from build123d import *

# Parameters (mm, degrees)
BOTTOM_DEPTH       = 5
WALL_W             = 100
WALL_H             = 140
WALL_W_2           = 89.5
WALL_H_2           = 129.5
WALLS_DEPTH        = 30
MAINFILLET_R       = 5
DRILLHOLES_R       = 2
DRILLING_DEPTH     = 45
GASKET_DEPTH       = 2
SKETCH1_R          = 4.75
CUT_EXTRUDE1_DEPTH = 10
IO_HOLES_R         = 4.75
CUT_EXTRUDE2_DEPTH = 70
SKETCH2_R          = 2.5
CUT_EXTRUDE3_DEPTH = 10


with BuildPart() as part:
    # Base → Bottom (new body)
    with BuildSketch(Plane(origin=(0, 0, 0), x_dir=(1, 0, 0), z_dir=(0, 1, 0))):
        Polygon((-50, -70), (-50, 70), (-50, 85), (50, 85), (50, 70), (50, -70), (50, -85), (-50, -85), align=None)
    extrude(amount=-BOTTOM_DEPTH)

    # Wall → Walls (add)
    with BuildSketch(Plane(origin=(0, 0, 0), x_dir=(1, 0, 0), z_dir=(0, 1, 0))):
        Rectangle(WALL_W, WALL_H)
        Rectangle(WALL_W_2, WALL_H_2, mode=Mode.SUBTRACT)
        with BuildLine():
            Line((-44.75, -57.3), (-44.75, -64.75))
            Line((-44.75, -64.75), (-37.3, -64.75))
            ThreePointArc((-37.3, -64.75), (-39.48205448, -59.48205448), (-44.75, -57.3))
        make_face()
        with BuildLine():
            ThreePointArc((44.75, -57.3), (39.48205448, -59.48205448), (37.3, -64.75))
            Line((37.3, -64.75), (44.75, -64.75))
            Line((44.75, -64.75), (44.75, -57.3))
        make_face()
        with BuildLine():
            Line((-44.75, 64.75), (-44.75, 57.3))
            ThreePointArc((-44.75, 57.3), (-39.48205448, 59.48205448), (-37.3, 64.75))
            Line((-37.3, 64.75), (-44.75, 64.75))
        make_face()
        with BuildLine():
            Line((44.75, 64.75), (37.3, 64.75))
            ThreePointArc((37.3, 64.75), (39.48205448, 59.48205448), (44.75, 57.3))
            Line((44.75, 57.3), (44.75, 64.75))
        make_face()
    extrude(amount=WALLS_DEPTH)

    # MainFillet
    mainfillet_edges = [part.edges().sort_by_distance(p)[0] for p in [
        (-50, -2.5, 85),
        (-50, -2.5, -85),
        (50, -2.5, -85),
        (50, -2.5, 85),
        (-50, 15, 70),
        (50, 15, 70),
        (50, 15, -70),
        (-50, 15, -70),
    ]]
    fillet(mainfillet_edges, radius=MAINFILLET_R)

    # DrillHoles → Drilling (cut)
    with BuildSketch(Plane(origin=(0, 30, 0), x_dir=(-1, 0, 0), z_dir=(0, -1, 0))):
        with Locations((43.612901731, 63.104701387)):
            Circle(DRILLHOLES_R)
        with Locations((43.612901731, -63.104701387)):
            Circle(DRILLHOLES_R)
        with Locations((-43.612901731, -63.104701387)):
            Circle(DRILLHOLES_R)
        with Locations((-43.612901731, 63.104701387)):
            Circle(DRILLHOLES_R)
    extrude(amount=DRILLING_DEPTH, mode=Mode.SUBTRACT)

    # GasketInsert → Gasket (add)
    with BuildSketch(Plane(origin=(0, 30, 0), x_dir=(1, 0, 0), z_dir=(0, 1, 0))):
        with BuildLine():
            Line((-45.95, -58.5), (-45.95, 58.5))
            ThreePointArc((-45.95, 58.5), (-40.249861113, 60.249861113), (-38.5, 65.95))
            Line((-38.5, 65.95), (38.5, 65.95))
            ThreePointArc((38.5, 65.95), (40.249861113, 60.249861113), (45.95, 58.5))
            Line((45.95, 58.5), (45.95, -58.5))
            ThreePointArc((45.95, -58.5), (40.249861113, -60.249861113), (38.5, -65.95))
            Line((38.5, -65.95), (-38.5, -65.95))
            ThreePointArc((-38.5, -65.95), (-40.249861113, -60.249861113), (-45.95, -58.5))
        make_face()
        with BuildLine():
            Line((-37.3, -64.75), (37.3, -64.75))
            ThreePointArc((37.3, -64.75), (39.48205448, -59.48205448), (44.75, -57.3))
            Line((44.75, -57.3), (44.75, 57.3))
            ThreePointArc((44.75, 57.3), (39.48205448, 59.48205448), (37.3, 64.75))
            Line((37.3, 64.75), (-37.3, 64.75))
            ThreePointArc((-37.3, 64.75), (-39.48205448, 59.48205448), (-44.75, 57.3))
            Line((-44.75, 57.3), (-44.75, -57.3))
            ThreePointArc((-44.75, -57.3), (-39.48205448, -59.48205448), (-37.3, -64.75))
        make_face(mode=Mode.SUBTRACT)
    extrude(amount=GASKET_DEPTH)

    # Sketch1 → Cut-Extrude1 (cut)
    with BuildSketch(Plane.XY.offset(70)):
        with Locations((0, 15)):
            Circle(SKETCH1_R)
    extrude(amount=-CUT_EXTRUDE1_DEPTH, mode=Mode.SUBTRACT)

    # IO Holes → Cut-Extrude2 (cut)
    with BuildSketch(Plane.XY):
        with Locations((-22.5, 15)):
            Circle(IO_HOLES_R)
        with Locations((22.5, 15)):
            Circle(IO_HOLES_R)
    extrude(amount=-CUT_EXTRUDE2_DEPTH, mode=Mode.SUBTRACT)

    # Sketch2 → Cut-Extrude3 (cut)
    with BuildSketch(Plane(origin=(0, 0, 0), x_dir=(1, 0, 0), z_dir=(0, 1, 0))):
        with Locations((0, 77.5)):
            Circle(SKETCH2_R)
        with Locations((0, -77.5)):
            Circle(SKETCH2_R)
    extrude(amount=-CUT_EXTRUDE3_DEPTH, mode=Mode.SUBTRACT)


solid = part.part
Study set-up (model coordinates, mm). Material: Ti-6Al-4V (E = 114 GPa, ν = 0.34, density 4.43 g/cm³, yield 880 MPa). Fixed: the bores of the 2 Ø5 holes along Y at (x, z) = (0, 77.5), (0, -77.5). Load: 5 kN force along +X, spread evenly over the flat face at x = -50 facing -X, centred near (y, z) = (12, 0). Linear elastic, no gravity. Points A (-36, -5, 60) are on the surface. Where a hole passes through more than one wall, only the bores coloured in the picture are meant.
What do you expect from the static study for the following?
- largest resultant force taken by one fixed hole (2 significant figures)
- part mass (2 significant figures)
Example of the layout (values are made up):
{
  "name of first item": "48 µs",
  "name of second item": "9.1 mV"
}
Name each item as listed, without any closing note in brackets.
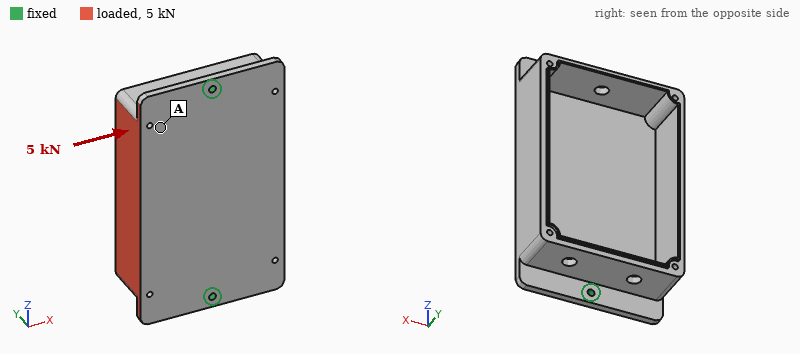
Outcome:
{
  "largest resultant force taken by one fixed hole": "2.5 kN",
  "part mass": "710 g"
}
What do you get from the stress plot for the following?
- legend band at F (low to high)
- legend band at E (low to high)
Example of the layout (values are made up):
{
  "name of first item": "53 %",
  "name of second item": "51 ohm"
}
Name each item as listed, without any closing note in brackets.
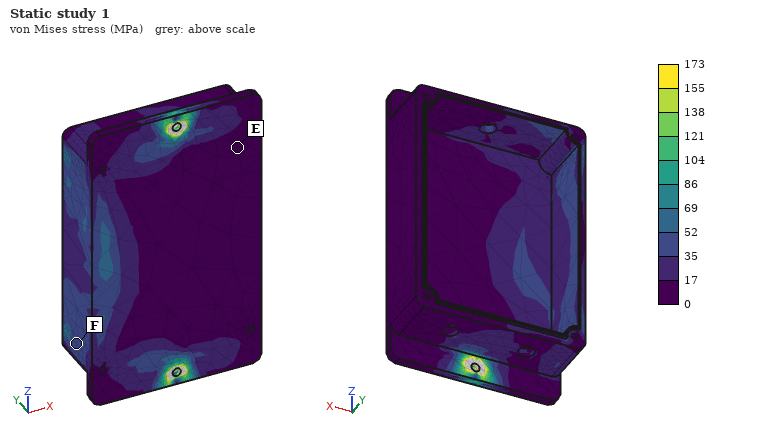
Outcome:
{
  "legend band at F": "35 to 52 MPa",
  "legend band at E": "0 to 17 MPa"
}
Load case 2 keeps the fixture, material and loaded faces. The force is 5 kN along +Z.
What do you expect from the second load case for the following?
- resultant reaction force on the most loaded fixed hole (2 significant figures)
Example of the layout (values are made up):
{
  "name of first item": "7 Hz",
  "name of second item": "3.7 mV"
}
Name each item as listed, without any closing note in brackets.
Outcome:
{
  "resultant reaction force on the most loaded fixed hole": "3.0 kN"
}
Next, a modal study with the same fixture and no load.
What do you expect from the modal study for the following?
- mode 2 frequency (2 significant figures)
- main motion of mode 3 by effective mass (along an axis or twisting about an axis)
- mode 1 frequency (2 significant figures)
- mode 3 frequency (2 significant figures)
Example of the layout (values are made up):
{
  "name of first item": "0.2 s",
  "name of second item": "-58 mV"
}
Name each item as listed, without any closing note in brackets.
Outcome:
{
  "mode 2 frequency": "1300 Hz",
  "main motion of mode 3 by effective mass": "along Y",
  "mode 1 frequency": "600 Hz",
  "mode 3 frequency": "1900 Hz"
}
